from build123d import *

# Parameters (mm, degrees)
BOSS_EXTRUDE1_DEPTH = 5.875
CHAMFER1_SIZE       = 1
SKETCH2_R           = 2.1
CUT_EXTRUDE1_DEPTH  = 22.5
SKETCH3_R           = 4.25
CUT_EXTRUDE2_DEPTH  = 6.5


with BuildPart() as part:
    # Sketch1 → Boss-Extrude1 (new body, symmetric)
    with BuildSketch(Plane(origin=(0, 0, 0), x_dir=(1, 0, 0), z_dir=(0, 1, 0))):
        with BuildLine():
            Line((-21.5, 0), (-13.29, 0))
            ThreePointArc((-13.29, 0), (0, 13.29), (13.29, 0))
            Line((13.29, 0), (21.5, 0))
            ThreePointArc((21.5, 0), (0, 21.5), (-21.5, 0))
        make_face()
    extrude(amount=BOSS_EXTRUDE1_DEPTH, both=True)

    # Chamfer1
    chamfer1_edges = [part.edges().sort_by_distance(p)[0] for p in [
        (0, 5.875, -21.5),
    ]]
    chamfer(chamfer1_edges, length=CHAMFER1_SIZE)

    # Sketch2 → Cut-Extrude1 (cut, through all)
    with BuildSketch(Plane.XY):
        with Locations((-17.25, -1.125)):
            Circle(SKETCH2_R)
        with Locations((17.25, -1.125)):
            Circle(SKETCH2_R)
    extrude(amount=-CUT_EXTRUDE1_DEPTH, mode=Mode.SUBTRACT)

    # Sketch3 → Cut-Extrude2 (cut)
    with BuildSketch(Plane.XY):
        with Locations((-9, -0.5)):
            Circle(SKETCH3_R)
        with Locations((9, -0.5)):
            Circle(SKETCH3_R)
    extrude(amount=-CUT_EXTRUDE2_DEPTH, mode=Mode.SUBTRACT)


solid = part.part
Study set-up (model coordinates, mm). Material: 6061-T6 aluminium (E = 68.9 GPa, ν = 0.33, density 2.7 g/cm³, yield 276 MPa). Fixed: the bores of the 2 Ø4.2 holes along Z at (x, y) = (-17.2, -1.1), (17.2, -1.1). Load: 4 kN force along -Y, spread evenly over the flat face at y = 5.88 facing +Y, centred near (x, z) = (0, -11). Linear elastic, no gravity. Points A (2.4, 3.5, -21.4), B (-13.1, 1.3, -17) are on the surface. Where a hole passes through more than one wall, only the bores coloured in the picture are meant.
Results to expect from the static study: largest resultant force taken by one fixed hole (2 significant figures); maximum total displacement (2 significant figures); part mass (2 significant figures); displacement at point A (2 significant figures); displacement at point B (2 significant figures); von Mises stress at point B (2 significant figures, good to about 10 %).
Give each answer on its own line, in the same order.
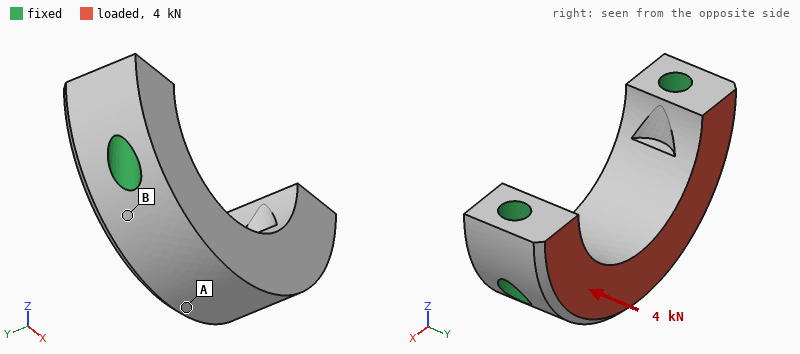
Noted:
2.0 kN
18 µm
13 g
18 µm
6.4 µm
35 MPa
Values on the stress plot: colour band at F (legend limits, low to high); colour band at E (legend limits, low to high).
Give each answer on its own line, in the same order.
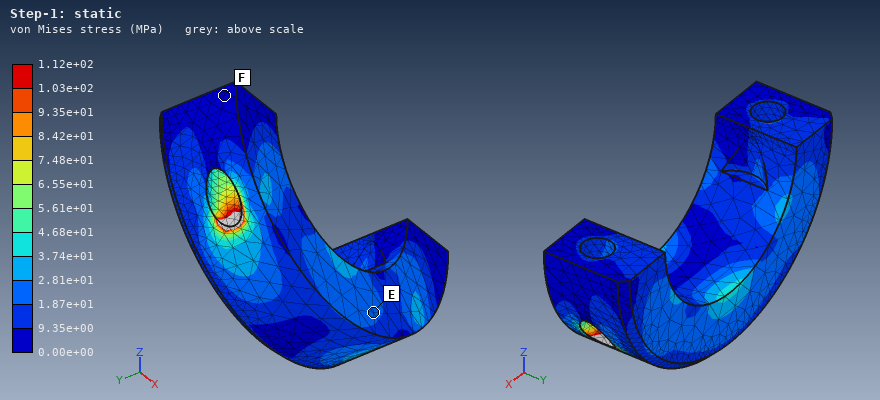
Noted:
0.00e+00 to 9.35e+00 MPa
1.87e+01 to 2.81e+01 MPa
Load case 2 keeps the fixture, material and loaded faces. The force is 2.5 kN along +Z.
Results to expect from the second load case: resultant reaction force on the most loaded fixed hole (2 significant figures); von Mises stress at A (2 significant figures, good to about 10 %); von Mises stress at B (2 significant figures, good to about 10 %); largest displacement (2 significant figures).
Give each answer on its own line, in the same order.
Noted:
1.3 kN
17 MPa
20 MPa
14 µm
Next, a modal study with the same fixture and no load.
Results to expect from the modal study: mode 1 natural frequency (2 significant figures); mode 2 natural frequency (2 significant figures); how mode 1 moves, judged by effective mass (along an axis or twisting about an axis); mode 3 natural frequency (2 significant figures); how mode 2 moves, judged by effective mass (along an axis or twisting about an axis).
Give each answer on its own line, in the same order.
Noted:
24 kHz
39 kHz
along Y
50 kHz
along Z
